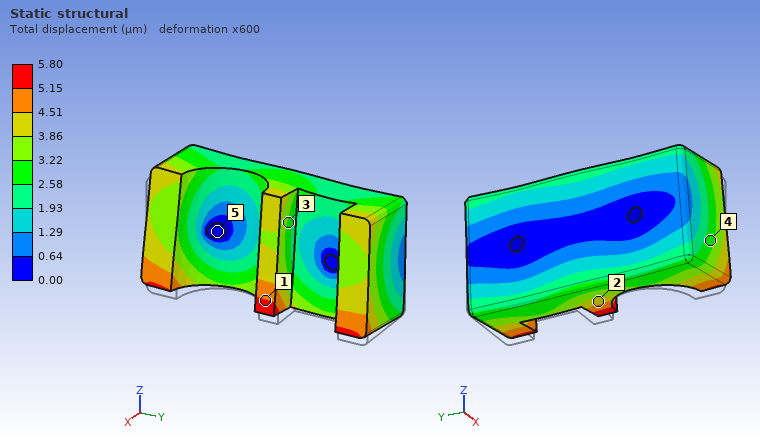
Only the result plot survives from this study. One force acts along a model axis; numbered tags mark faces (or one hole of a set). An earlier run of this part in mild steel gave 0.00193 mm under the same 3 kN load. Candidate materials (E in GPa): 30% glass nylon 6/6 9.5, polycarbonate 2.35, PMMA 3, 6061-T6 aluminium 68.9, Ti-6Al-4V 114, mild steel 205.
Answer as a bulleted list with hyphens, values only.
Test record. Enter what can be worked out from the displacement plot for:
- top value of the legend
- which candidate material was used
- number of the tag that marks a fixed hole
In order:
- 5.80 µm
- 6061-T6 aluminium
- 5
